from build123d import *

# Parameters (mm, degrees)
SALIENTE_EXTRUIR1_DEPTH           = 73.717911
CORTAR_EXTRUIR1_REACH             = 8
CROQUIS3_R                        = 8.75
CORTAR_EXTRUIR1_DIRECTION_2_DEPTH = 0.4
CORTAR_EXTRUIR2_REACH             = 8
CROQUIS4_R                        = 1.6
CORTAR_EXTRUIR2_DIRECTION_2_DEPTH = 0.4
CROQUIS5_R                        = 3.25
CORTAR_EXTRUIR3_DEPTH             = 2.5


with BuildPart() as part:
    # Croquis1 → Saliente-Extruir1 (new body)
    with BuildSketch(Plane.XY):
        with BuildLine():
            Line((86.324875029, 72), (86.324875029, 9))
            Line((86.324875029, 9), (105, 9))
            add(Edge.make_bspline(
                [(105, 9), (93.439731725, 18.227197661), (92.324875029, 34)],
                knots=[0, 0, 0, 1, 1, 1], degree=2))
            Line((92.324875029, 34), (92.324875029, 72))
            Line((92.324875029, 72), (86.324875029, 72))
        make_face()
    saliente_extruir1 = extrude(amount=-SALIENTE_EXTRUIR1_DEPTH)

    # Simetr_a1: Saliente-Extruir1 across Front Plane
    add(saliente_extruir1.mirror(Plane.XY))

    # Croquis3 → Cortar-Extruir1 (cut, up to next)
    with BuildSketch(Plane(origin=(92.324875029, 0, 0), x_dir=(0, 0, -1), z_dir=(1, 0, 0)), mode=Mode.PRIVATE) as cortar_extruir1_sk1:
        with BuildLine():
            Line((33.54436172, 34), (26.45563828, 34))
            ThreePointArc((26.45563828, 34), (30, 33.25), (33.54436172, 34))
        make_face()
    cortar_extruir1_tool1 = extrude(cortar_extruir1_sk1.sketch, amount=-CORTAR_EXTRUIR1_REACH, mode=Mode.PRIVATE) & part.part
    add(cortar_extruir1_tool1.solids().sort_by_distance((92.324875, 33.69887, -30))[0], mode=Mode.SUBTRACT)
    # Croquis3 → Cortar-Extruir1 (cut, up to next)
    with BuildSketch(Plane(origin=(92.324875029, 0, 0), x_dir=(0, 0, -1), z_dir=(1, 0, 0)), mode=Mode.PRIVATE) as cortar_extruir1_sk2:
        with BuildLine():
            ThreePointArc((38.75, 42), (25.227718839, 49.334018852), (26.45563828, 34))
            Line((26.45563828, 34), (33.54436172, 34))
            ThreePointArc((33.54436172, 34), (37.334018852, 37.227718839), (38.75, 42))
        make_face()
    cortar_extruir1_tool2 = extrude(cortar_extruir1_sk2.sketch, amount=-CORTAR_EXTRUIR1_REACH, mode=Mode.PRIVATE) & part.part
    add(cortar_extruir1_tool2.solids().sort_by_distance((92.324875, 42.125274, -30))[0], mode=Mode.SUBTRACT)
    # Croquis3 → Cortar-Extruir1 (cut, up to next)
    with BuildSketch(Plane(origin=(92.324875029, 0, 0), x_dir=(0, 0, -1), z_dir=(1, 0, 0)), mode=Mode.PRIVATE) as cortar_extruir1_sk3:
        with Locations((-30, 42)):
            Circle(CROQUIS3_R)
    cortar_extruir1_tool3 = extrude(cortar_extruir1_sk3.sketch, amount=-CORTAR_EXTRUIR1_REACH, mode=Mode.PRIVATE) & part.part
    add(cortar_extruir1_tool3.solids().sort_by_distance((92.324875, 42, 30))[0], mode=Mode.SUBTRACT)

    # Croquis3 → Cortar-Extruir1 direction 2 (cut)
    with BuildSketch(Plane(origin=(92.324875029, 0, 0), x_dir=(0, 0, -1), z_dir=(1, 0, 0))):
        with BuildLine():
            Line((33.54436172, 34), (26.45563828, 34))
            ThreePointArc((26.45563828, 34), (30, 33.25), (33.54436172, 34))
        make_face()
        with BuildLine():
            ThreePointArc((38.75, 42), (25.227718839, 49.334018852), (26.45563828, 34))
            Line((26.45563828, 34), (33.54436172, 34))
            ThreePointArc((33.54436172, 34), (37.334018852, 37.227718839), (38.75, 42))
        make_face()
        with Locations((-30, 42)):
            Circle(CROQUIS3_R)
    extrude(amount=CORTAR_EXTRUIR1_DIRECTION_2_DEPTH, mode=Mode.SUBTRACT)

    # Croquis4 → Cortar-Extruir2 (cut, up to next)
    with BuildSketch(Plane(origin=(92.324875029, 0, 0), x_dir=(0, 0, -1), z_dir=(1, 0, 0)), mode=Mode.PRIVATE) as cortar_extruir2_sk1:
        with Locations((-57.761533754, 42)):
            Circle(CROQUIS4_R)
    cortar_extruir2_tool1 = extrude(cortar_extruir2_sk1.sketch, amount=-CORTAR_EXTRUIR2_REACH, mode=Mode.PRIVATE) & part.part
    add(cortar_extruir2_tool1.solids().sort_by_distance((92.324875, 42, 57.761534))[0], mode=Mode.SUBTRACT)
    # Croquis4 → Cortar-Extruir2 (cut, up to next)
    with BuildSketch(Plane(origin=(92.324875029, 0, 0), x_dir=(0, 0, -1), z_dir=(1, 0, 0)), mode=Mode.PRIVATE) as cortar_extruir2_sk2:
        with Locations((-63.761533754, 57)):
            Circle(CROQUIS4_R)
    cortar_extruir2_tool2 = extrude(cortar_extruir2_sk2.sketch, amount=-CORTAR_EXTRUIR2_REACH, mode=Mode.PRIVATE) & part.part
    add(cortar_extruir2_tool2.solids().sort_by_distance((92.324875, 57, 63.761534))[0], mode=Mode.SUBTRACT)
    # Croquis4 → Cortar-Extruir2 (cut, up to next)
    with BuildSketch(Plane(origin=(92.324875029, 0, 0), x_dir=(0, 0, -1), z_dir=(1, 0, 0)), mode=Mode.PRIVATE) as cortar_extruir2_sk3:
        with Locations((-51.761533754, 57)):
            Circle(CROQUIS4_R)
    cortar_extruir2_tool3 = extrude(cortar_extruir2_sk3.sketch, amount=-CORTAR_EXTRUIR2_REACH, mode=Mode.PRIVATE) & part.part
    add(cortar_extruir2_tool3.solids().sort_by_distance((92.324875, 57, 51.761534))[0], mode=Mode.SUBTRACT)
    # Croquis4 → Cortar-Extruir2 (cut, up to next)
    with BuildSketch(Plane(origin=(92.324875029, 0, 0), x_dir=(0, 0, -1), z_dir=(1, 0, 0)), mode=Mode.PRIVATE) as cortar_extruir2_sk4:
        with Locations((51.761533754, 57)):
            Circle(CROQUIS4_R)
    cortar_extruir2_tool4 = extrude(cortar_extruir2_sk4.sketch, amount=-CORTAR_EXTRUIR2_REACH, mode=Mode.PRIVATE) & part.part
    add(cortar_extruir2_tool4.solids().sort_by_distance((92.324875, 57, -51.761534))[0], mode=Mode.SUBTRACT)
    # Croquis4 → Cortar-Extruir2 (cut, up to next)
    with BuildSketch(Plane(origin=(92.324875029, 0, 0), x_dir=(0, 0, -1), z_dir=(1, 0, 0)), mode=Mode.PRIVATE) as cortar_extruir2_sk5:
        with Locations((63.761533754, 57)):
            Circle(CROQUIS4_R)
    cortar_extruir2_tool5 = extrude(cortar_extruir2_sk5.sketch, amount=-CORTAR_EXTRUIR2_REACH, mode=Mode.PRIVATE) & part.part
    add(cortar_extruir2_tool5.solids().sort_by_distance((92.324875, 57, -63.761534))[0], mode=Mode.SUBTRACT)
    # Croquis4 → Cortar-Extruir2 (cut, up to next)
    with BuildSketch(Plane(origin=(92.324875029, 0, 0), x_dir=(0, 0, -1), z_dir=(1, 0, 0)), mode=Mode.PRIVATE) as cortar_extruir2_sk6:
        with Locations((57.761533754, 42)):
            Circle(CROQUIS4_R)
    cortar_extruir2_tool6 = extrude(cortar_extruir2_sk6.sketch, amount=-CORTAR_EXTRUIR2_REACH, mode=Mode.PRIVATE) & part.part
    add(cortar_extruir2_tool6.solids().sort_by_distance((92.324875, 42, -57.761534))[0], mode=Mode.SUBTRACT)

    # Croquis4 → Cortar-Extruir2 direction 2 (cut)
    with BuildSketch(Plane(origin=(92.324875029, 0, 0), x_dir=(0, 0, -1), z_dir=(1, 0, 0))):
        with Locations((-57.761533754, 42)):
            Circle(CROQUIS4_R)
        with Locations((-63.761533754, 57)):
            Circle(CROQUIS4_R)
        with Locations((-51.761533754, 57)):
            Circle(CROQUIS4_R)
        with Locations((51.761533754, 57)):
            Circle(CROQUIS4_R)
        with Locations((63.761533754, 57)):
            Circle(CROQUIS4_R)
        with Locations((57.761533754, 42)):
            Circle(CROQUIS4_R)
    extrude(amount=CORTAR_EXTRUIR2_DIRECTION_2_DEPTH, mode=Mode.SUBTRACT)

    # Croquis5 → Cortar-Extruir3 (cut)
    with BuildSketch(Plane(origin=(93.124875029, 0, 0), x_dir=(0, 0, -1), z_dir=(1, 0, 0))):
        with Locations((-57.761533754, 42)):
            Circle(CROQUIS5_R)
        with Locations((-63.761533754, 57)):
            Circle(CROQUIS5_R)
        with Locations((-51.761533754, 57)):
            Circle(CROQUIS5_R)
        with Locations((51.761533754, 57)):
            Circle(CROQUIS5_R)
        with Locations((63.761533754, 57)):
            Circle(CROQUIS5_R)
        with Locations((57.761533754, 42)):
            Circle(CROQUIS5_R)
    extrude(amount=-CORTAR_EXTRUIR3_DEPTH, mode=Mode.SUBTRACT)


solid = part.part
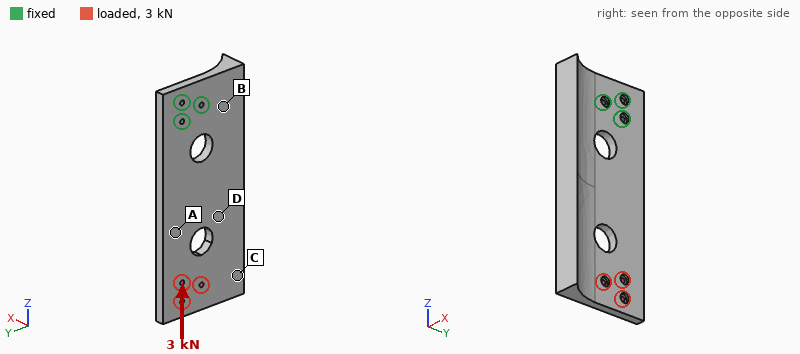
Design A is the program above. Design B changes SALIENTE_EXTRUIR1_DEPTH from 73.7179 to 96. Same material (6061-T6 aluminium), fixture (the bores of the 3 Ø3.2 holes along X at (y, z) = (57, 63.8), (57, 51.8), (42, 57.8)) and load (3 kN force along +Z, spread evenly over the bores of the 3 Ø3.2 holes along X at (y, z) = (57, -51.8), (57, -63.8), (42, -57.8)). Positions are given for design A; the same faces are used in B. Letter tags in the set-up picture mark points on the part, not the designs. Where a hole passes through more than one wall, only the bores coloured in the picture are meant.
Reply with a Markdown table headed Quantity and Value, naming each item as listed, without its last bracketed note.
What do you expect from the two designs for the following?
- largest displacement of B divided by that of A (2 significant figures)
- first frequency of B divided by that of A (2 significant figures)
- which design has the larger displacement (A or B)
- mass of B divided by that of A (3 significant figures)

| Quantity | Value |
|---|---|
| largest displacement of B divided by that of A | 1.2 |
| first frequency of B divided by that of A | 0.81 |
| which design has the larger displacement | B |
| mass of B divided by that of A | 1.32 |
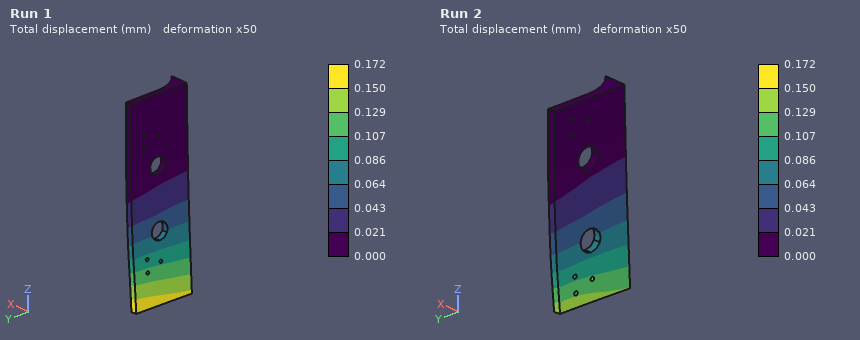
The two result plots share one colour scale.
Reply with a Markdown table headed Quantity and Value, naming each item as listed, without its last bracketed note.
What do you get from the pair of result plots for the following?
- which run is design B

| Quantity | Value |
|---|---|
| which run is design B | Run 1 |
